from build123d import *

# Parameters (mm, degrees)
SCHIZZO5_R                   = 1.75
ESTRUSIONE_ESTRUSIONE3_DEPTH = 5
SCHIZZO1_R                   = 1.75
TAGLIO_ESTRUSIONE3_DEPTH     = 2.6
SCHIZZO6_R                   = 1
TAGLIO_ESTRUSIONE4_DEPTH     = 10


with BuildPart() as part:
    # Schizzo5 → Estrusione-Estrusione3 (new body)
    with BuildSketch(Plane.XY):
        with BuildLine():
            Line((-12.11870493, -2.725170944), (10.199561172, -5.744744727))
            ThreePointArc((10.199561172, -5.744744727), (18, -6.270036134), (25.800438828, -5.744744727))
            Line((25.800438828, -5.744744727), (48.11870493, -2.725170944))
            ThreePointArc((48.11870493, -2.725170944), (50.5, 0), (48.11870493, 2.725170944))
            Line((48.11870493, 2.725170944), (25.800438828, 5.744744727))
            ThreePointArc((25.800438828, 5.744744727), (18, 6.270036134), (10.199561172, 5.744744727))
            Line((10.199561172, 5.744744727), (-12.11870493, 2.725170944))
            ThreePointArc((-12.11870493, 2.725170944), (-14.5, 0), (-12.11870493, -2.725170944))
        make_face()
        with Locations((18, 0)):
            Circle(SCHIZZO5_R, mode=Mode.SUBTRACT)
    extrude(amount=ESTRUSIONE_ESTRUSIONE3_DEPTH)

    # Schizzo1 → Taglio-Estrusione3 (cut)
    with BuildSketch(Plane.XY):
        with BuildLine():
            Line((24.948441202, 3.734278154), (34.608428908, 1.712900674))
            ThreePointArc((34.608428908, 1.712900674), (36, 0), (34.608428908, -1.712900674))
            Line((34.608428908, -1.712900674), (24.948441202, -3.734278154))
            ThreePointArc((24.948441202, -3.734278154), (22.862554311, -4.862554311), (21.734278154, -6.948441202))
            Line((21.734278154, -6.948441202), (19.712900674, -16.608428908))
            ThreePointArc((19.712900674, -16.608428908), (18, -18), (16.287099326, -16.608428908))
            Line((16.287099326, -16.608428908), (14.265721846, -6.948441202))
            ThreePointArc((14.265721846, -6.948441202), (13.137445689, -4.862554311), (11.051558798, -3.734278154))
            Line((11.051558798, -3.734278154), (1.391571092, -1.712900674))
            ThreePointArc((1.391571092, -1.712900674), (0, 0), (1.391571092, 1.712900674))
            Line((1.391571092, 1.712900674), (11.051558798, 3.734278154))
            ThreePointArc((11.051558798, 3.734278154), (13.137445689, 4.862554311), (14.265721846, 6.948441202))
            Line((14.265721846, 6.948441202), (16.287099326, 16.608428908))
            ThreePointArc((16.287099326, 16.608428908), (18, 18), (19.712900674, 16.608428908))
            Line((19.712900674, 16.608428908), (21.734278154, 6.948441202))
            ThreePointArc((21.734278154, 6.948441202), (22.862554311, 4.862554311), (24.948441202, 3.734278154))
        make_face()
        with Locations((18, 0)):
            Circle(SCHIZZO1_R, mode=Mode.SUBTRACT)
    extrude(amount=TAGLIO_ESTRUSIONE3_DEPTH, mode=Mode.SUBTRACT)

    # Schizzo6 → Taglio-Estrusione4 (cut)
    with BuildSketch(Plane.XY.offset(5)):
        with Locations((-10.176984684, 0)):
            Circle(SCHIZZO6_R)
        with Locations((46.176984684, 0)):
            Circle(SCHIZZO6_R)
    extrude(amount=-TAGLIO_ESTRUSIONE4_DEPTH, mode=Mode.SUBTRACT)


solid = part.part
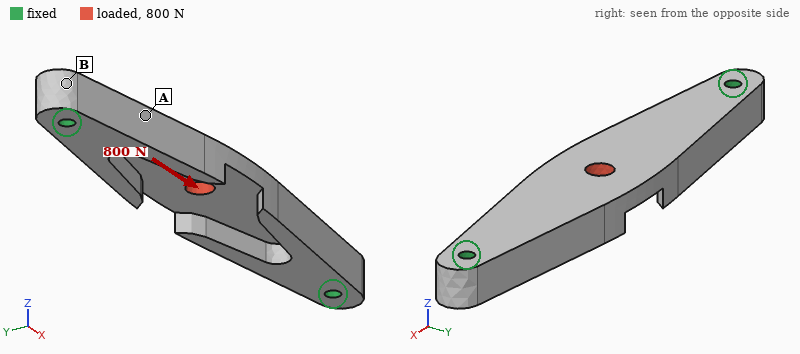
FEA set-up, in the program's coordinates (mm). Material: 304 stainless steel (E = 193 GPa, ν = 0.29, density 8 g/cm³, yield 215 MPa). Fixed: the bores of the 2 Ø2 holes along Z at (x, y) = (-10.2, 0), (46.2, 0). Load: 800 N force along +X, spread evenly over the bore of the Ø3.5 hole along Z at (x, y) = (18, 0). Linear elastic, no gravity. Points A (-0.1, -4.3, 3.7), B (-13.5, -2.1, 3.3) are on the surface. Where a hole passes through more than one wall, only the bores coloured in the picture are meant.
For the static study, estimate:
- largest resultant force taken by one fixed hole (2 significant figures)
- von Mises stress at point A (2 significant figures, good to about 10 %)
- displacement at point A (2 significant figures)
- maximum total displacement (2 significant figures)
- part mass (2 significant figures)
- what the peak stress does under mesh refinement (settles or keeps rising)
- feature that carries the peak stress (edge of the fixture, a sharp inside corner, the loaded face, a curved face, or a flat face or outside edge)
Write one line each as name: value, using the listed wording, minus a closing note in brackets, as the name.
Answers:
largest resultant force taken by one fixed hole: 400 N
von Mises stress at point A: 12 MPa
displacement at point A: 0.69 µm
maximum total displacement: 2.2 µm
part mass: 18 g
what the peak stress does under mesh refinement: keeps rising
feature that carries the peak stress: a sharp inside corner
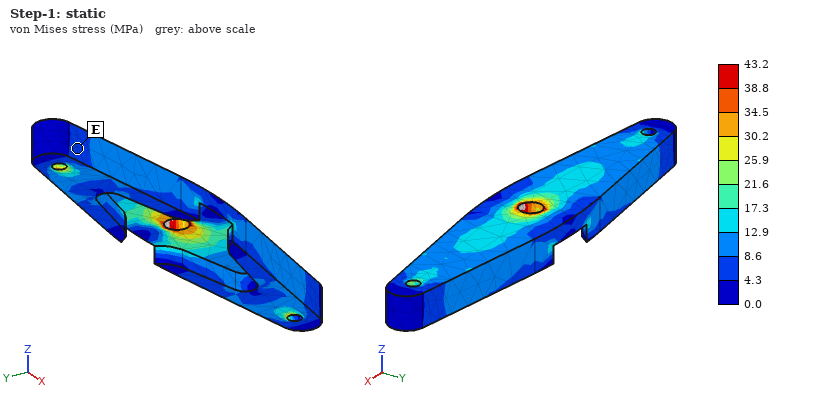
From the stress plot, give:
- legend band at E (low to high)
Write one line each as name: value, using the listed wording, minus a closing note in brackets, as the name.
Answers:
legend band at E: 4.3 to 8.6 MPa
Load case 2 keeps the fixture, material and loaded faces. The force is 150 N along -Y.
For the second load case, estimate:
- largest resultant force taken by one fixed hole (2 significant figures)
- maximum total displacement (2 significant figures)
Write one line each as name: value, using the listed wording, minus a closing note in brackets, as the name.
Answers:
largest resultant force taken by one fixed hole: 75 N
maximum total displacement: 5.5 µm
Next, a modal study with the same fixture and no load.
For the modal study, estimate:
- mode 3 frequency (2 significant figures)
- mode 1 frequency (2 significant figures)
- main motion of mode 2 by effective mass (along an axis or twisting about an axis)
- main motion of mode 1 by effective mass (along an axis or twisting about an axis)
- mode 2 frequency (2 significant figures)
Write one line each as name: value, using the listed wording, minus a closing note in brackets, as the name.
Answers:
mode 3 frequency: 15 kHz
mode 1 frequency: 6500 Hz
main motion of mode 2 by effective mass: along Y
main motion of mode 1 by effective mass: along Z
mode 2 frequency: 10 kHz
